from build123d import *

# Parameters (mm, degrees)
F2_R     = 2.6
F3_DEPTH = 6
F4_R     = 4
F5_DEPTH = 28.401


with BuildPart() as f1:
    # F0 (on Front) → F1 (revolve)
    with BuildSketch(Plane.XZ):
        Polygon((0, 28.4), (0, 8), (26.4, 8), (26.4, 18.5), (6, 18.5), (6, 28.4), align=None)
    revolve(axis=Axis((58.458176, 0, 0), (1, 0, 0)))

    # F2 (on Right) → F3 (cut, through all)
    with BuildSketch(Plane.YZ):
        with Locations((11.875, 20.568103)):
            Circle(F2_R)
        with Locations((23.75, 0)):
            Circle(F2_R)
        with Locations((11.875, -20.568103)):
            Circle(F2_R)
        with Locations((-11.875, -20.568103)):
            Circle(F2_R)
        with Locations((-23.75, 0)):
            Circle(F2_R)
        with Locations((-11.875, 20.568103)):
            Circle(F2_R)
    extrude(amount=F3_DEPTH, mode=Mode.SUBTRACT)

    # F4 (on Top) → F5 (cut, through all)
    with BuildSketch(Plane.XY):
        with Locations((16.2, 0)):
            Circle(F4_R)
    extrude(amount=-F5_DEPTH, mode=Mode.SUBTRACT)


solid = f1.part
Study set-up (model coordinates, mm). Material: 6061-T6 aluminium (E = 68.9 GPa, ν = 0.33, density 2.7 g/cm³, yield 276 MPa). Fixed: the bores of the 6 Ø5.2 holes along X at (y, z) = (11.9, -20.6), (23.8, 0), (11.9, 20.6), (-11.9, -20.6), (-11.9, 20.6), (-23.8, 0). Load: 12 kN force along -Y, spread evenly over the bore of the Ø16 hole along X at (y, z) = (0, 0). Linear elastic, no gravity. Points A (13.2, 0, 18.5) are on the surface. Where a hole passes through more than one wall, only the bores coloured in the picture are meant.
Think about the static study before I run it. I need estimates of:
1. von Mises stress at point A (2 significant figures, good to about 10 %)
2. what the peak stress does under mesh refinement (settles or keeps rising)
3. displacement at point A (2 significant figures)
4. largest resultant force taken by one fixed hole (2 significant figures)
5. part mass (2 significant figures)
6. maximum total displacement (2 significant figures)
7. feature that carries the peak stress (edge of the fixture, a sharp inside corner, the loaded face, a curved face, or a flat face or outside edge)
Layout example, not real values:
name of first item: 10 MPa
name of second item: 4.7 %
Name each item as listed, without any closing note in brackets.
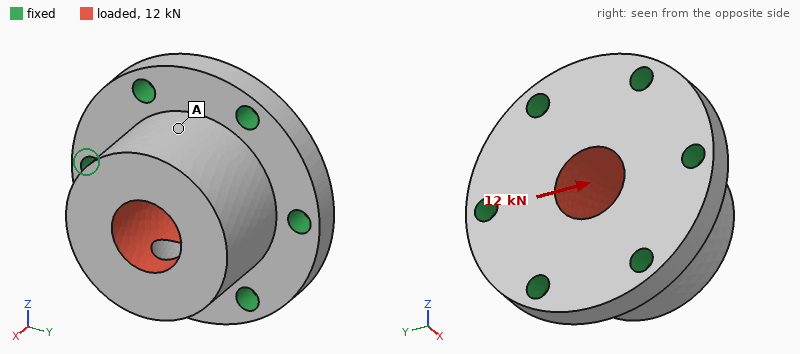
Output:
von Mises stress at point A: 13 MPa
what the peak stress does under mesh refinement: keeps rising
displacement at point A: 9.6 µm
largest resultant force taken by one fixed hole: 3.4 kN
part mass: 82 g
maximum total displacement: 23 µm
feature that carries the peak stress: edge of the fixture
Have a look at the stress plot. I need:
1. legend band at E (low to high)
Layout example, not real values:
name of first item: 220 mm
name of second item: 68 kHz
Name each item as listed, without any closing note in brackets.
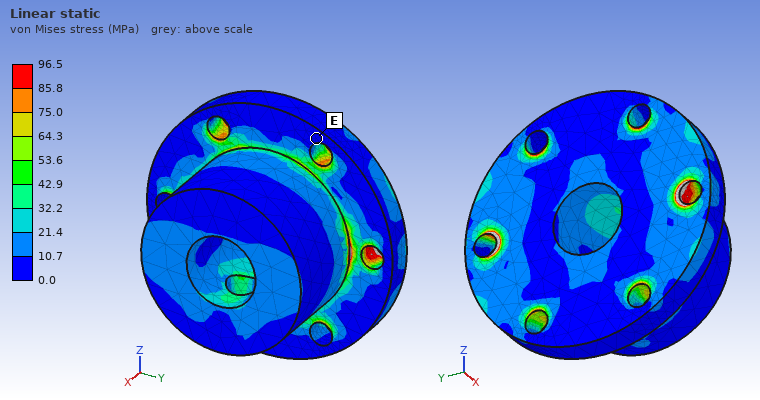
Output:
legend band at E: 0.0 to 10.7 MPa
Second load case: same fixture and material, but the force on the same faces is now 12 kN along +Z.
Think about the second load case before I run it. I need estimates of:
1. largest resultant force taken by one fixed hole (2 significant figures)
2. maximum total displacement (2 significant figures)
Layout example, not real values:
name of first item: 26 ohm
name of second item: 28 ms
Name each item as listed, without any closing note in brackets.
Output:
largest resultant force taken by one fixed hole: 3.0 kN
maximum total displacement: 22 µm
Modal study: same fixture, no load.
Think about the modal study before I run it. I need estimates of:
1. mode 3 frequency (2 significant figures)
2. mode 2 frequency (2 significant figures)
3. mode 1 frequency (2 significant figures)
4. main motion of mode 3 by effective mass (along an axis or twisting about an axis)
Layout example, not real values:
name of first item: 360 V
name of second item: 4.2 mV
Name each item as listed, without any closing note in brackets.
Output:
mode 3 frequency: 21 kHz
mode 2 frequency: 17 kHz
mode 1 frequency: 17 kHz
main motion of mode 3 by effective mass: along X
